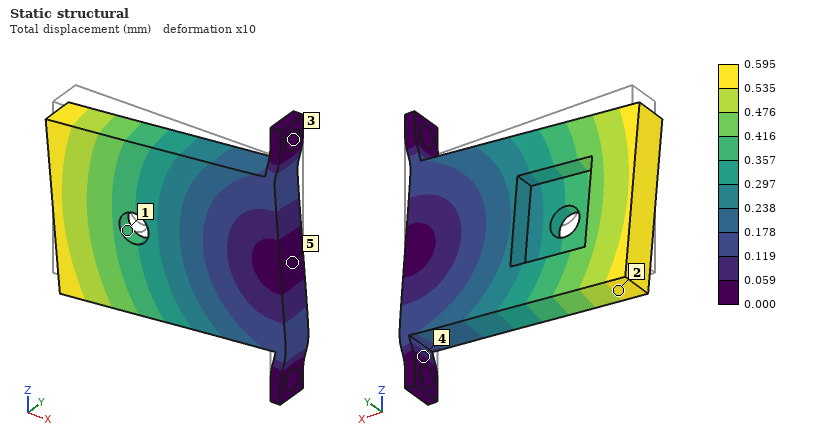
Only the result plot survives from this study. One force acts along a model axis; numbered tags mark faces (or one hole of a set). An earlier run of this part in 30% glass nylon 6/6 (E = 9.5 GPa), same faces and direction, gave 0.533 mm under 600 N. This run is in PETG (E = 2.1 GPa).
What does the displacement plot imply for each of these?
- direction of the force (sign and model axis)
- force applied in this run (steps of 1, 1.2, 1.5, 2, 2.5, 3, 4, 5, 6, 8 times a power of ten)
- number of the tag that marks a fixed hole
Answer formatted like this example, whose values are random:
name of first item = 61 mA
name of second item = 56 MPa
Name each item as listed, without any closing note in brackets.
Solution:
direction of the force = -Z
force applied in this run = 150 N
number of the tag that marks a fixed hole = 3
